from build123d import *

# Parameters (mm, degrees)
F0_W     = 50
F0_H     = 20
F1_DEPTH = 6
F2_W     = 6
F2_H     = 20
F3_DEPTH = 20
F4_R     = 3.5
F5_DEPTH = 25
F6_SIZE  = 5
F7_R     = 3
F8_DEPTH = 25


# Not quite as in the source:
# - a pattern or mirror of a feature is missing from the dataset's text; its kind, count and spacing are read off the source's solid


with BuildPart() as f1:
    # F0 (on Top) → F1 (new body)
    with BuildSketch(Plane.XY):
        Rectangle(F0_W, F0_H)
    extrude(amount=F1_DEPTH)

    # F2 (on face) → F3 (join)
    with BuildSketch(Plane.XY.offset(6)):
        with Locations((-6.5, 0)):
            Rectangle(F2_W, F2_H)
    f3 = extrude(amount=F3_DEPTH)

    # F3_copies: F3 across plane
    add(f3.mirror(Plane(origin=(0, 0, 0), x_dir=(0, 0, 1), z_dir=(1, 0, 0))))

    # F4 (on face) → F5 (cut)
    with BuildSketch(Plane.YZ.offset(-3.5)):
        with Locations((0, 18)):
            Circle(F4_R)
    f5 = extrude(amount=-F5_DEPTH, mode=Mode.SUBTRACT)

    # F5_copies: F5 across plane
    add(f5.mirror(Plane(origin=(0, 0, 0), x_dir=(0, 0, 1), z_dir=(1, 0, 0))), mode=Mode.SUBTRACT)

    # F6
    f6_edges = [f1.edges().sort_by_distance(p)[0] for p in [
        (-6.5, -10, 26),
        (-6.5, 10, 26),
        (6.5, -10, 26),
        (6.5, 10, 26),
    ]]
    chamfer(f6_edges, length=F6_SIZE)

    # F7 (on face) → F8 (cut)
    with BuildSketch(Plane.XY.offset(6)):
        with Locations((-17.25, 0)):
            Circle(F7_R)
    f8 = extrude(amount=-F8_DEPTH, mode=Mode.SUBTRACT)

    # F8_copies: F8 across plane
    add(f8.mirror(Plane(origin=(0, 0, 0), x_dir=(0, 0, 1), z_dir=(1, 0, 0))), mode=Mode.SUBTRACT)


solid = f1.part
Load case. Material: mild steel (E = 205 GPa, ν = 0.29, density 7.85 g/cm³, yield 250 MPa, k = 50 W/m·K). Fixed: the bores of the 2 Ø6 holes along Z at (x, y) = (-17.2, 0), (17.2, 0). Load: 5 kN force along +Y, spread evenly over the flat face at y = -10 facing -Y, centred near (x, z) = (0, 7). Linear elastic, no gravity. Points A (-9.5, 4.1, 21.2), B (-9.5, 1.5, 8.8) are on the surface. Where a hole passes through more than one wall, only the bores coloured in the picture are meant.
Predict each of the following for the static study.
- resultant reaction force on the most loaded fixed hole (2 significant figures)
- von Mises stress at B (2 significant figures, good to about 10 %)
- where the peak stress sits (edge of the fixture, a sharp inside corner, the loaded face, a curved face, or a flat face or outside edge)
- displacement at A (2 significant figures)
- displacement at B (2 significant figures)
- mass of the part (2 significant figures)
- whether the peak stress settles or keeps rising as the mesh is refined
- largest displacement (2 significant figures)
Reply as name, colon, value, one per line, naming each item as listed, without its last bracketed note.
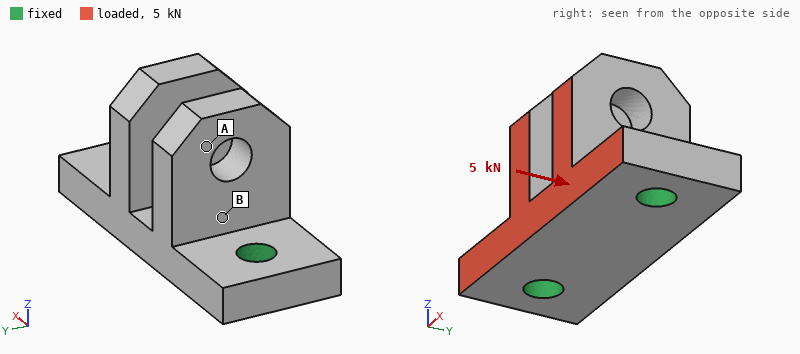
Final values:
resultant reaction force on the most loaded fixed hole: 2.5 kN
von Mises stress at B: 31 MPa
where the peak stress sits: edge of the fixture
displacement at A: 17 µm
displacement at B: 6.7 µm
mass of the part: 76 g
whether the peak stress settles or keeps rising as the mesh is refined: keeps rising
largest displacement: 21 µm
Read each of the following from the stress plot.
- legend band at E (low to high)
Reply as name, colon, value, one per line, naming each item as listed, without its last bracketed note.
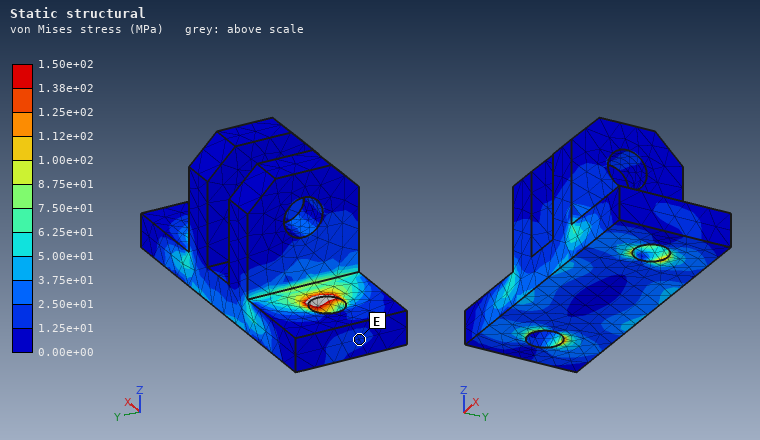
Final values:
legend band at E: 1.25e+01 to 2.50e+01 MPa
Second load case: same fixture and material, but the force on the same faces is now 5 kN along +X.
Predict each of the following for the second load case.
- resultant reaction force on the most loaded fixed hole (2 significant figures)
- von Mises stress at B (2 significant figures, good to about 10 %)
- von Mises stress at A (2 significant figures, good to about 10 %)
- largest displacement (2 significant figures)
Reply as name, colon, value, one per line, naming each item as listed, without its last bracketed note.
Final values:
resultant reaction force on the most loaded fixed hole: 2.9 kN
von Mises stress at B: 44 MPa
von Mises stress at A: 23 MPa
largest displacement: 20 µm
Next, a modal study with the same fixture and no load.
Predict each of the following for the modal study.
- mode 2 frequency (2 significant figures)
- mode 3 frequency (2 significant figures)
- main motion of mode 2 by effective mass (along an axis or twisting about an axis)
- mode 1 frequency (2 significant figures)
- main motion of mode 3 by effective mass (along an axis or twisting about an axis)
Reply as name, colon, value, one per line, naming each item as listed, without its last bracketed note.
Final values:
mode 2 frequency: 9100 Hz
mode 3 frequency: 11 kHz
main motion of mode 2 by effective mass: along Y
mode 1 frequency: 8700 Hz
main motion of mode 3 by effective mass: along X
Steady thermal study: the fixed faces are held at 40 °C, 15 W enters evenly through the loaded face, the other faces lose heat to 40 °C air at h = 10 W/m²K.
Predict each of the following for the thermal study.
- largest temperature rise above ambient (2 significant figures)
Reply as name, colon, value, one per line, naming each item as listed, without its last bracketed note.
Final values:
largest temperature rise above ambient: 16 K
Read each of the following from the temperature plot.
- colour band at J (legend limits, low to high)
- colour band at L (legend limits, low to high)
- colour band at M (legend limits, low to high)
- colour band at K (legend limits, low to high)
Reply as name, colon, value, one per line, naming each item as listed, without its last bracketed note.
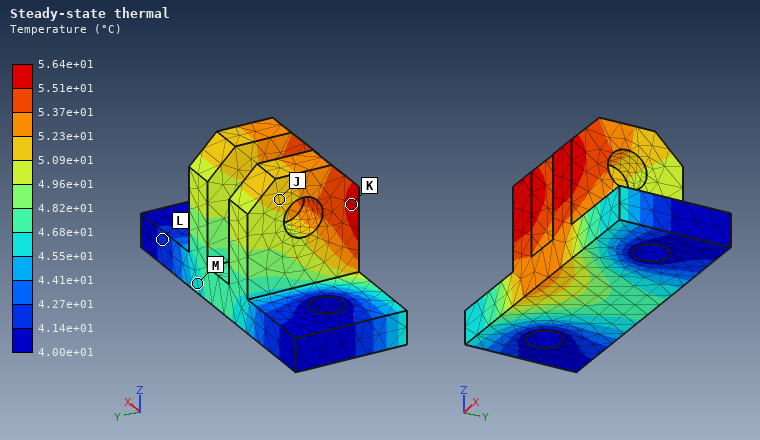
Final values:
colour band at J: 5.09e+01 to 5.23e+01 °C
colour band at L: 4.14e+01 to 4.27e+01 °C
colour band at M: 4.55e+01 to 4.68e+01 °C
colour band at K: 5.51e+01 to 5.64e+01 °C
